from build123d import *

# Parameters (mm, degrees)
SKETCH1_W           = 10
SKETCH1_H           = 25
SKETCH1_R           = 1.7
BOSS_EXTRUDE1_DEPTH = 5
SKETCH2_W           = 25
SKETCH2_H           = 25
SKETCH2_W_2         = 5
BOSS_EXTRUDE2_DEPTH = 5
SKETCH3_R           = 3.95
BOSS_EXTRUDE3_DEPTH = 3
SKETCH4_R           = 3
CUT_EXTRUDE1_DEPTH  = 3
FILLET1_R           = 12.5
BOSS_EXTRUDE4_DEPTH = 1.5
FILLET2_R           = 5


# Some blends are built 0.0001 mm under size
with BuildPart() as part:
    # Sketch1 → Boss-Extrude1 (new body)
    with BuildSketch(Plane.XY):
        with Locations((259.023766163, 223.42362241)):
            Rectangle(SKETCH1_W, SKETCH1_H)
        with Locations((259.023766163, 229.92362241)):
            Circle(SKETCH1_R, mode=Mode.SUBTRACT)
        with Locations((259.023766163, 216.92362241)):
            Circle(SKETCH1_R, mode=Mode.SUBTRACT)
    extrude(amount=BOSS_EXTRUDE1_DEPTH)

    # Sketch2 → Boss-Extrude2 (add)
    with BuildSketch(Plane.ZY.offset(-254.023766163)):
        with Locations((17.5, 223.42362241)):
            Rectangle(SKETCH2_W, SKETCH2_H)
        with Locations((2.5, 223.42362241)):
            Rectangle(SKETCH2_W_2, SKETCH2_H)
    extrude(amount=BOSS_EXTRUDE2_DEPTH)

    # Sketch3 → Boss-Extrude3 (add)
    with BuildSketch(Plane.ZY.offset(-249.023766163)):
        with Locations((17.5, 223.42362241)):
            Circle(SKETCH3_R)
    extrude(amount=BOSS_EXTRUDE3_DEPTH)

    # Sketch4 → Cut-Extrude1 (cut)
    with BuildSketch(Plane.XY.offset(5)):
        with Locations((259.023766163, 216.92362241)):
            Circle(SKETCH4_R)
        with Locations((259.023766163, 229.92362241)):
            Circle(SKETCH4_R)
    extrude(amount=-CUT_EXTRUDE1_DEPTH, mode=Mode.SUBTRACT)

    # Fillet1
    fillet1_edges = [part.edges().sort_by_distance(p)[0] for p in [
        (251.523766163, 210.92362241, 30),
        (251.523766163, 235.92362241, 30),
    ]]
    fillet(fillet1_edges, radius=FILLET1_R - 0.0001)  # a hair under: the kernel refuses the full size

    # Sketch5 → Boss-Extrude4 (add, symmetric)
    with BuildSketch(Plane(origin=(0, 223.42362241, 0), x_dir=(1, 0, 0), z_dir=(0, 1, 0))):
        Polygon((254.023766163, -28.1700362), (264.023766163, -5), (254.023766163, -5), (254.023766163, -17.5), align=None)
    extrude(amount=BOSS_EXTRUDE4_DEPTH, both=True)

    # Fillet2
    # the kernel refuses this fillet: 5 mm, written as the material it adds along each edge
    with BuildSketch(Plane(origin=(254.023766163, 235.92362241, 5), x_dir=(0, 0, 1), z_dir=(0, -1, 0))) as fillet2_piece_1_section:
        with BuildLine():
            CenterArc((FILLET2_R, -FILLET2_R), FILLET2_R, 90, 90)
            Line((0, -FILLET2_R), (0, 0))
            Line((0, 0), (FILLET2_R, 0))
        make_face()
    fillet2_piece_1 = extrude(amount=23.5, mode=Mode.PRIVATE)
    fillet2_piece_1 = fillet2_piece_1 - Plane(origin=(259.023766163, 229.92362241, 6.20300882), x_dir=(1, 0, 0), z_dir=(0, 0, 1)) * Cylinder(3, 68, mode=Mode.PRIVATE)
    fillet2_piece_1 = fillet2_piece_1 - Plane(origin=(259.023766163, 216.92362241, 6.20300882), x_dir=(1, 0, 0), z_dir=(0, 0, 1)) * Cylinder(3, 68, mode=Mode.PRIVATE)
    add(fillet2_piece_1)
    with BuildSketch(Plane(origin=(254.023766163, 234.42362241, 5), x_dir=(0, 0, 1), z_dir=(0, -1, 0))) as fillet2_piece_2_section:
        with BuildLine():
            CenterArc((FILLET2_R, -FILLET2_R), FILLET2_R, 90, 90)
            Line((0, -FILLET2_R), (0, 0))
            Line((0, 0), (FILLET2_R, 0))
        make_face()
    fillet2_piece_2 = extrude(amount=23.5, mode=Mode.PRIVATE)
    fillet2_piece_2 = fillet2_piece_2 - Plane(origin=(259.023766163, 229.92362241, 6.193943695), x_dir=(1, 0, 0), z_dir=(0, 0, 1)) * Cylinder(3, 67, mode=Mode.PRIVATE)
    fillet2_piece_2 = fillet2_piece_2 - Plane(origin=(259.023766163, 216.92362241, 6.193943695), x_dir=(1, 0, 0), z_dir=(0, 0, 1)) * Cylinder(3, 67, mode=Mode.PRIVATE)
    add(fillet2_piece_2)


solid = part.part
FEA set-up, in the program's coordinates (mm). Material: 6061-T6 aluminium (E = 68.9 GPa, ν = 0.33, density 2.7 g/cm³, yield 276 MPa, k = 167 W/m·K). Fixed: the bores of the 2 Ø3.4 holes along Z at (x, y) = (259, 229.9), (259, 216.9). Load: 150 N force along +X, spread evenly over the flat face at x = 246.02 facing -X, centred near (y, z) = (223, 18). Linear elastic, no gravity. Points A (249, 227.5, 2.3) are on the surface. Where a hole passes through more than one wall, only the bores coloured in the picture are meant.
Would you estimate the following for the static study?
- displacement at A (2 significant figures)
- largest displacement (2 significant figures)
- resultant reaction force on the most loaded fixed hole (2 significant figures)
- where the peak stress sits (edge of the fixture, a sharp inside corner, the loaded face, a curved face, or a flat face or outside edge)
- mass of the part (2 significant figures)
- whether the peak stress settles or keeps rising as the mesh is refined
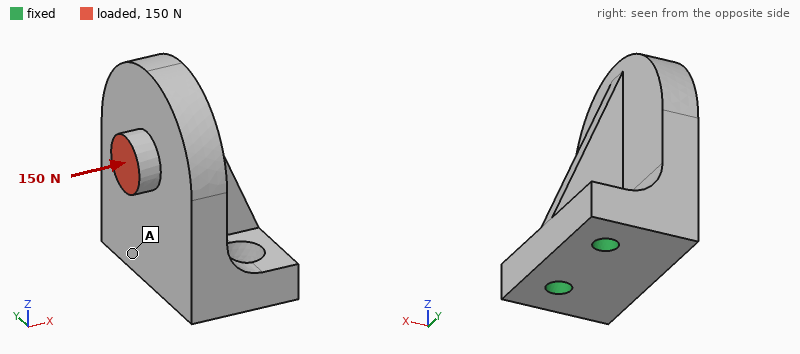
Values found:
14 µm
49 µm
82 N
edge of the fixture
14 g
keeps rising
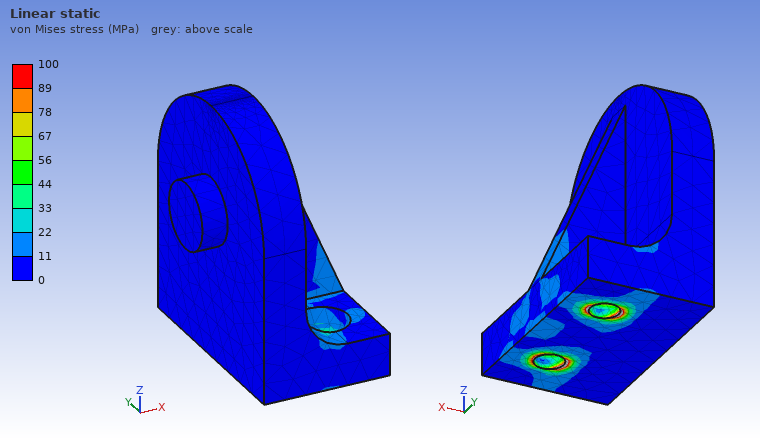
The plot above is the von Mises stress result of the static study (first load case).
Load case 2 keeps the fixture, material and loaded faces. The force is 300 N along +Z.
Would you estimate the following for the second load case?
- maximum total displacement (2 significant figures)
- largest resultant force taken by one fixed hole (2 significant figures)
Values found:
76 µm
150 N
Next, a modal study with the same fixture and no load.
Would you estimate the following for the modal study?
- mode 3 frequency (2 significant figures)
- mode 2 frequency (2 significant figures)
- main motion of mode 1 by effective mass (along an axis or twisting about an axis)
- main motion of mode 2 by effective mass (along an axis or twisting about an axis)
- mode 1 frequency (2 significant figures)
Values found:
16 kHz
8300 Hz
along X
along Y
3700 Hz
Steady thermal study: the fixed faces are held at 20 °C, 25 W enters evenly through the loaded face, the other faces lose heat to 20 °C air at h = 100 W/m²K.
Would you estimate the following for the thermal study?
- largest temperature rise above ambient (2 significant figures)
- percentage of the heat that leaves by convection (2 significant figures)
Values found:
35 K
14 %
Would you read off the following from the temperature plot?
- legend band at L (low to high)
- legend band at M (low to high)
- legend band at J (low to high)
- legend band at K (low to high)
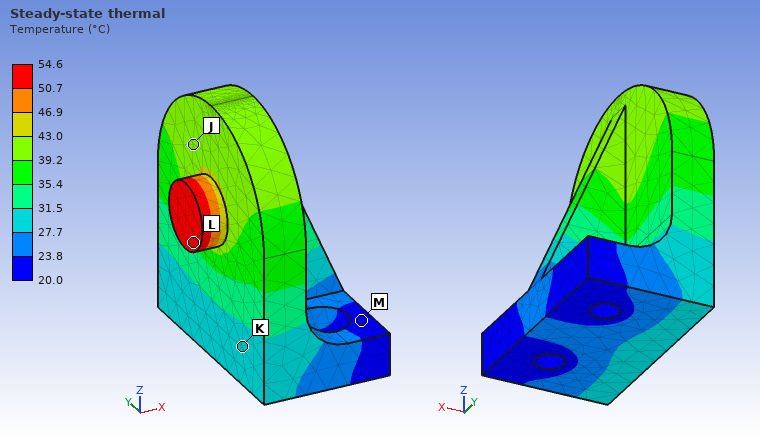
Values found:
50.7 to 54.6 °C
20.0 to 23.8 °C
39.2 to 43.0 °C
27.7 to 31.5 °C
